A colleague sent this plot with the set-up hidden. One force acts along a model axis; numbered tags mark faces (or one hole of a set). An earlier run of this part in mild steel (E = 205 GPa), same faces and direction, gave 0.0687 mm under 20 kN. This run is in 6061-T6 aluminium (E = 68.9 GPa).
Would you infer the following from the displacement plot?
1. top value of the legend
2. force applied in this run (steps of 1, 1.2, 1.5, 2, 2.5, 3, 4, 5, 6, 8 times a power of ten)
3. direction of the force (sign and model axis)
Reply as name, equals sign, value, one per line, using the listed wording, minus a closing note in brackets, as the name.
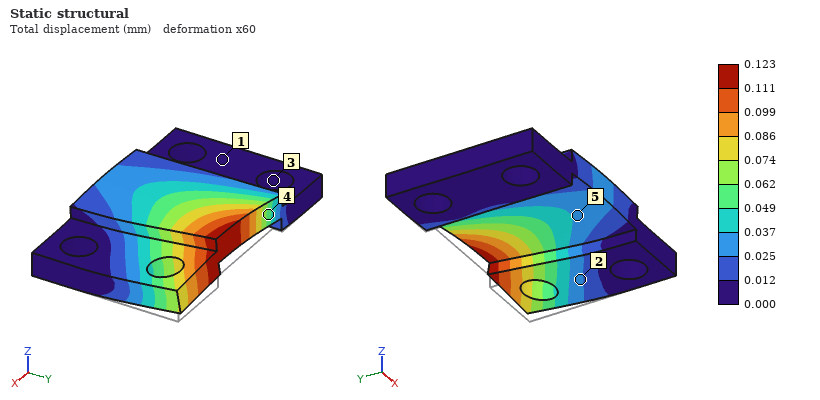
top value of the legend = 0.123 mm
force applied in this run = 12 kN
direction of the force = +Z
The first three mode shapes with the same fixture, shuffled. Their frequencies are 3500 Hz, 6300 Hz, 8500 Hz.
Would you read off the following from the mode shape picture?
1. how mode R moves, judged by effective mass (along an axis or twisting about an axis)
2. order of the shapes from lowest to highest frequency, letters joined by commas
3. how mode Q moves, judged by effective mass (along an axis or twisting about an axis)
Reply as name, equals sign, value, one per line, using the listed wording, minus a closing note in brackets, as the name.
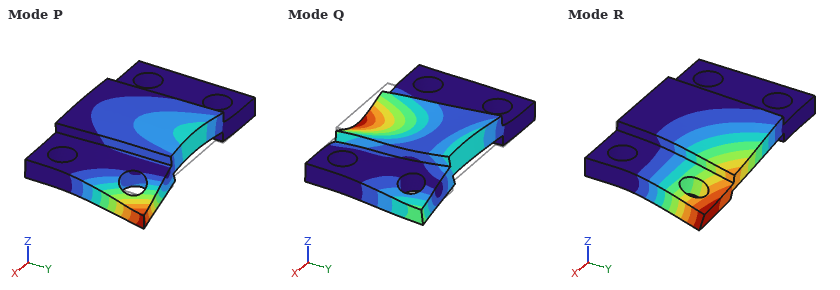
how mode R moves, judged by effective mass = along Z
order of the shapes from lowest to highest frequency, letters joined by commas = R, P, Q
how mode Q moves, judged by effective mass = along Z
